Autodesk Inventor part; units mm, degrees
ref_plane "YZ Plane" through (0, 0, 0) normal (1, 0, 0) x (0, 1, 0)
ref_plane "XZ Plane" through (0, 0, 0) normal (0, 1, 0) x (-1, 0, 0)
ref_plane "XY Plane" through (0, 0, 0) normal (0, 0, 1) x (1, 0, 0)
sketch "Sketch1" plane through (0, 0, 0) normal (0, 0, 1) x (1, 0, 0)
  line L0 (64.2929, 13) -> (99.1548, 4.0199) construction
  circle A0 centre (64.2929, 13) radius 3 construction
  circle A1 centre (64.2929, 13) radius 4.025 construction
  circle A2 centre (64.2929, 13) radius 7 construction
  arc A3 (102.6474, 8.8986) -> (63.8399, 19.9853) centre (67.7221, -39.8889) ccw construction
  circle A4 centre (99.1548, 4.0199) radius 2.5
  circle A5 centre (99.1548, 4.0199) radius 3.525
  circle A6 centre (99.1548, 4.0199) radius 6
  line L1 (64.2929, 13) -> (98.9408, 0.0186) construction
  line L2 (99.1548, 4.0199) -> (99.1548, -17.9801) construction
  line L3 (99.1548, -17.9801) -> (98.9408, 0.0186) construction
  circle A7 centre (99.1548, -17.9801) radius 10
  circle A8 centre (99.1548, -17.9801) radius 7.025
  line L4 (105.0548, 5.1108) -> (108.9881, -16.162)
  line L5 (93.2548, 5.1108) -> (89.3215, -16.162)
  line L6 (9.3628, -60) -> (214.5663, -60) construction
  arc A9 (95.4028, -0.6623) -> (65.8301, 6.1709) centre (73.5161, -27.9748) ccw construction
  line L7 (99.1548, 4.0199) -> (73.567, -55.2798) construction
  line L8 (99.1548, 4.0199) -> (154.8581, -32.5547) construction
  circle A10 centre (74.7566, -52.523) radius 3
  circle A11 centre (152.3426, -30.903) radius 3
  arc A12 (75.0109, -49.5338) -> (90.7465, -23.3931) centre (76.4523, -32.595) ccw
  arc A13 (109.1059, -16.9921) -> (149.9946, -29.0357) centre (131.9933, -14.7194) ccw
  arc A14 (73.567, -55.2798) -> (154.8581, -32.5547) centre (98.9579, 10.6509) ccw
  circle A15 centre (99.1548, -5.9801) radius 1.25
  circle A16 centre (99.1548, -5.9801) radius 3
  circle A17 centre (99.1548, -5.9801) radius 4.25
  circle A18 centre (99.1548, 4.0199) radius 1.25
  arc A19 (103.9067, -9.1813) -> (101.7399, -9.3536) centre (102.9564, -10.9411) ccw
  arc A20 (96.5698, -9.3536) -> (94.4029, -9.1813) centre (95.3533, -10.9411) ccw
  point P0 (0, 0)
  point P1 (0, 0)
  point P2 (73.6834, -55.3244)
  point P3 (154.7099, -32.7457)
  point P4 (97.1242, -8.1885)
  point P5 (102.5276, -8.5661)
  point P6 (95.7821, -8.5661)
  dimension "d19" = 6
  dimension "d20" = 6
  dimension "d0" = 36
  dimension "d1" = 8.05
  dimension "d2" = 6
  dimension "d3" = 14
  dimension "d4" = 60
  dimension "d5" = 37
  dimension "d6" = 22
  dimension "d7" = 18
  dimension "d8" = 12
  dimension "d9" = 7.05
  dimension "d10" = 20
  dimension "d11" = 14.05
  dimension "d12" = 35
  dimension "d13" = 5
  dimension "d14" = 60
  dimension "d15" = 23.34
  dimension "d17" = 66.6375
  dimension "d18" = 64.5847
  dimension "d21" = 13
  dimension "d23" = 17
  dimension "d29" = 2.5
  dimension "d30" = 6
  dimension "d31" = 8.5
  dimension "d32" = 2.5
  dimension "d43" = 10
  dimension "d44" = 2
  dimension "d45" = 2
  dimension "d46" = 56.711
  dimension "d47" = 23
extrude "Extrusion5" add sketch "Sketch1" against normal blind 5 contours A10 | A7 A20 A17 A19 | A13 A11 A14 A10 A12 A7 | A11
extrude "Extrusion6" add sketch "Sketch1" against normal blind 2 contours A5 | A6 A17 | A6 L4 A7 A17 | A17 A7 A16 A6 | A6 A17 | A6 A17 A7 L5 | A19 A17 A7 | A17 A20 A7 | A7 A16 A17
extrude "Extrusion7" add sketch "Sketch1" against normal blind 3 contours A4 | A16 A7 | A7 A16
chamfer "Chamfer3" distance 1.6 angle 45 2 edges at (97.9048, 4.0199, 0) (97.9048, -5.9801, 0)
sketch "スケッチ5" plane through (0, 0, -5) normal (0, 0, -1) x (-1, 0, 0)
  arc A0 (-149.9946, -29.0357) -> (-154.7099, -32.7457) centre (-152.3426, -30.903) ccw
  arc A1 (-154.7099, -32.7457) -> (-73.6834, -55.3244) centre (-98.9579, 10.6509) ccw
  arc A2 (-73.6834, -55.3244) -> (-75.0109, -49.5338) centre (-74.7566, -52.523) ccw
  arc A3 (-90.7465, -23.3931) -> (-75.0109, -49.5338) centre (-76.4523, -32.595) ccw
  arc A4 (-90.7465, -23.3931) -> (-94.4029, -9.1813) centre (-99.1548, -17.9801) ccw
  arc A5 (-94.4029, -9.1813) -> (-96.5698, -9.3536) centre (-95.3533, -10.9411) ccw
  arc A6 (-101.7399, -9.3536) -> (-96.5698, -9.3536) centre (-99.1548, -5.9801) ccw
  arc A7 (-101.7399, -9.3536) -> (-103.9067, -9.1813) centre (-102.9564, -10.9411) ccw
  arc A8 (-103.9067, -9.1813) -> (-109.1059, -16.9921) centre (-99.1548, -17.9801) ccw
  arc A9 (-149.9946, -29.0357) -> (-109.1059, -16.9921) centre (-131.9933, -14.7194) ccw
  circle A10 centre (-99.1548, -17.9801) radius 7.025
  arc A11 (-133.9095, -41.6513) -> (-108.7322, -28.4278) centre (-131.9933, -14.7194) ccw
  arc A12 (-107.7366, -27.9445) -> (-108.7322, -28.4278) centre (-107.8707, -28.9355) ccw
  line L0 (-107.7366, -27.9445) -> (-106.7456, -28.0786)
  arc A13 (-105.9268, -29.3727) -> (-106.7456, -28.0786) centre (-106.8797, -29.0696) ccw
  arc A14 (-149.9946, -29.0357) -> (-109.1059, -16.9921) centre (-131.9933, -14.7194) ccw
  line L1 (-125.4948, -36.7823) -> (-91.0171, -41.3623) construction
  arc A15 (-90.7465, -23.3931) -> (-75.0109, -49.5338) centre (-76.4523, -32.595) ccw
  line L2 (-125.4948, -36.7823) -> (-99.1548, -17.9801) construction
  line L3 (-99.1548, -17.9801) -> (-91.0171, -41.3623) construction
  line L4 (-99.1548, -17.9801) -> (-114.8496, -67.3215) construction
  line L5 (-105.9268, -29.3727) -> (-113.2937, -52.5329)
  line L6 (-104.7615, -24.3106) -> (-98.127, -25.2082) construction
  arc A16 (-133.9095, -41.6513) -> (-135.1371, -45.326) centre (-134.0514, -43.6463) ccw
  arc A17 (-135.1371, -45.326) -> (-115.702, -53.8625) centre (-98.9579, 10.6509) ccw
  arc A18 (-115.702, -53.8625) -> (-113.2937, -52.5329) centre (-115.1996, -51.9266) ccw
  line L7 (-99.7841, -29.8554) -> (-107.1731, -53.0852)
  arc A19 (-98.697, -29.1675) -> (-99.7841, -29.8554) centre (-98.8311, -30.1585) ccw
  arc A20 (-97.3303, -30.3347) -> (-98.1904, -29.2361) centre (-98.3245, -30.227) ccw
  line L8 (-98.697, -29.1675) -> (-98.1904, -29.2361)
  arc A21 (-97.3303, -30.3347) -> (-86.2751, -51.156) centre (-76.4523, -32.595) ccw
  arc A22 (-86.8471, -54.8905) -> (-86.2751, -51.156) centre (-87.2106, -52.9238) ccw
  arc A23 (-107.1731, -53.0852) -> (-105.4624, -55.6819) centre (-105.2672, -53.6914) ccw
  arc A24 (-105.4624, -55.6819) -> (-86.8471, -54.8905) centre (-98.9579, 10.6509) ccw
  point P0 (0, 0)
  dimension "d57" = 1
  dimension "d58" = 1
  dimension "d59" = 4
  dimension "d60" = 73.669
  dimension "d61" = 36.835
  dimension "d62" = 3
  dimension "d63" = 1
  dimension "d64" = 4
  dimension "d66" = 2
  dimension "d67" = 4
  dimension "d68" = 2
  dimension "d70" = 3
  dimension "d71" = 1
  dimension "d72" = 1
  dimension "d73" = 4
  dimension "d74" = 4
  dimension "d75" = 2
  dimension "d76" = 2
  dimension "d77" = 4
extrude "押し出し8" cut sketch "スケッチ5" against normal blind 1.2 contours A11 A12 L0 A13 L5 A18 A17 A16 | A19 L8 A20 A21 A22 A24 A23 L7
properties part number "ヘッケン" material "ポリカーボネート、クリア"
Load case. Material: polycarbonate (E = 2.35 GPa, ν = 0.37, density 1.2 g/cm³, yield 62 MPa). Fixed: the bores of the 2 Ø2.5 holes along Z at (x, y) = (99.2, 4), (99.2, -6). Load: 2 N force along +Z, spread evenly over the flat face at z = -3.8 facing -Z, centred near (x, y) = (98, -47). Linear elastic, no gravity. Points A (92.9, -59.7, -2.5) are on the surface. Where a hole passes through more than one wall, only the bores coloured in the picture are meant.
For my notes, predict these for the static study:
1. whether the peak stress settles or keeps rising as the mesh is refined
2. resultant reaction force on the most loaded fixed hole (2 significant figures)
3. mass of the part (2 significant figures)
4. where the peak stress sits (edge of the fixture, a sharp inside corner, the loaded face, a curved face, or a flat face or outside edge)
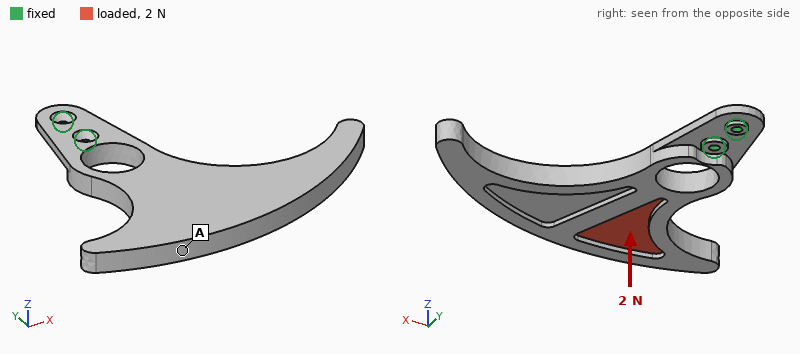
keeps rising
12 N
9.8 g
edge of the fixture
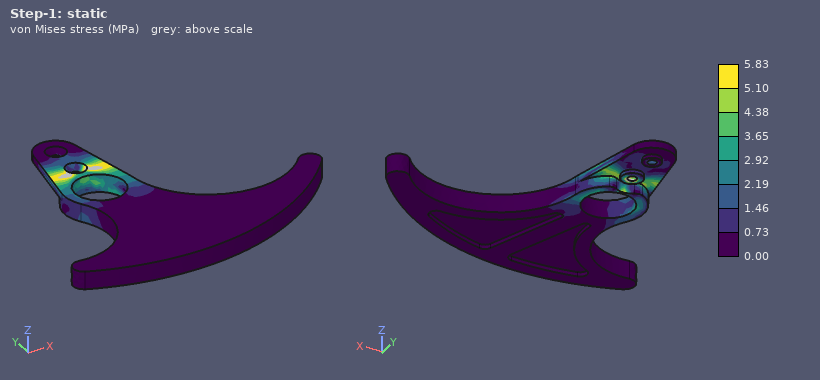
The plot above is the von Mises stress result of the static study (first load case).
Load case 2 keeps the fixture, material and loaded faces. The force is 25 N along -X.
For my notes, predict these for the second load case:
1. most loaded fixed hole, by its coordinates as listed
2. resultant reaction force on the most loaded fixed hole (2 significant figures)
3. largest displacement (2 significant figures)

(99.2, -6)
100 N
1.1 mm
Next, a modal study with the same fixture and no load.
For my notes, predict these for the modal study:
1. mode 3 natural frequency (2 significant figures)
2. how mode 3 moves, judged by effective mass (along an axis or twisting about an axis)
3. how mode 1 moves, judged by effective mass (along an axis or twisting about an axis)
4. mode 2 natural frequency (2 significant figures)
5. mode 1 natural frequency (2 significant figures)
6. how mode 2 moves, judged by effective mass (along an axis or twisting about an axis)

300 Hz
along X
along Z
160 Hz
85 Hz
twisting about Y
